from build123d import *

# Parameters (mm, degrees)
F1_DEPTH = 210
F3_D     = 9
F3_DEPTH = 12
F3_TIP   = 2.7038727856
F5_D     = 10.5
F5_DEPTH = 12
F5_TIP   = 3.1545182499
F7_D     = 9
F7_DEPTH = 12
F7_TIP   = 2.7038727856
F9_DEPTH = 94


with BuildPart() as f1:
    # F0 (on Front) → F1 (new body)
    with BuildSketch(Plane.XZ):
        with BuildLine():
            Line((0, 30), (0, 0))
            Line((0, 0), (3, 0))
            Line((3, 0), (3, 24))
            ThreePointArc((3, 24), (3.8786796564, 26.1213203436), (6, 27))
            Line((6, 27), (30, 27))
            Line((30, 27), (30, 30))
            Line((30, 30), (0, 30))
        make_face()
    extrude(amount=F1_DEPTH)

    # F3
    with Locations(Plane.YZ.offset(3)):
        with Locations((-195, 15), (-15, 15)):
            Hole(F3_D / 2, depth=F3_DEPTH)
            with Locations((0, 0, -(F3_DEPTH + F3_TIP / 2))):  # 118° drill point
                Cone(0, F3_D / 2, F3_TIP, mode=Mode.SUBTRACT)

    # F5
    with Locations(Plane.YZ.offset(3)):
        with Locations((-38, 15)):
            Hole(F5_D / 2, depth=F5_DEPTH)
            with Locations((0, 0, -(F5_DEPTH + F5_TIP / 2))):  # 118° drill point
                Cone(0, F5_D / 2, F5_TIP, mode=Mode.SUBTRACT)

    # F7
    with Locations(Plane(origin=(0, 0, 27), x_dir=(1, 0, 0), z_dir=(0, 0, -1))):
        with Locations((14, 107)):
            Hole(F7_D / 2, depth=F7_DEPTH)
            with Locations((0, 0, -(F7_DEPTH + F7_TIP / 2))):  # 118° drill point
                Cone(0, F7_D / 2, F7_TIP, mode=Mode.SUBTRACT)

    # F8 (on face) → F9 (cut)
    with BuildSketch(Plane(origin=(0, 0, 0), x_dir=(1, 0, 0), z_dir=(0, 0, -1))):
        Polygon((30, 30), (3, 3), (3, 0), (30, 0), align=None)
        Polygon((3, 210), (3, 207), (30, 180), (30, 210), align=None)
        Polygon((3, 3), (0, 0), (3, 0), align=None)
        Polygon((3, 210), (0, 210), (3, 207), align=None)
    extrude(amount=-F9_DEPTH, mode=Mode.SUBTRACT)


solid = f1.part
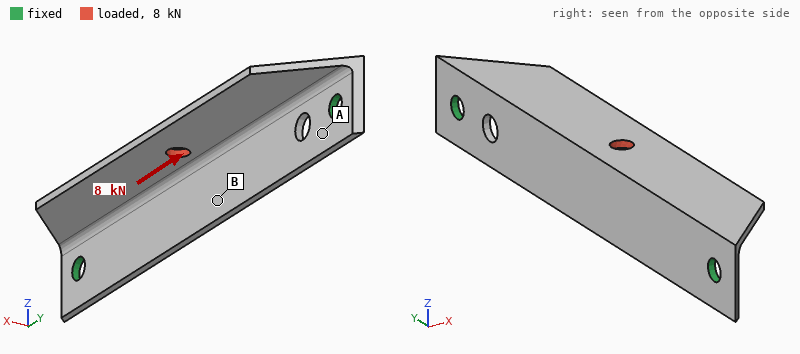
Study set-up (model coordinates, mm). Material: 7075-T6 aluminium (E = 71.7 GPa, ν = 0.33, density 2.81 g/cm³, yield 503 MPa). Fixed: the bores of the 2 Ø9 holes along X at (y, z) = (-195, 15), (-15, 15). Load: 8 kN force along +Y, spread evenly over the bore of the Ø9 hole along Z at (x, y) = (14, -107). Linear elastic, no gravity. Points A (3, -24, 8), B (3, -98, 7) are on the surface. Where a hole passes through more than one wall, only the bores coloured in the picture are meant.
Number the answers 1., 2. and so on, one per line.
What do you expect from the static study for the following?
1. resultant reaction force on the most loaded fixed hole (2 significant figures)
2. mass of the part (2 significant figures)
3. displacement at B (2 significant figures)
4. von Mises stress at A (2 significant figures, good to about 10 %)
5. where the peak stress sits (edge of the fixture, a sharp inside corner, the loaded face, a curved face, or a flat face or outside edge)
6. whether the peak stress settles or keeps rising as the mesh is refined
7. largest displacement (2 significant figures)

1. 4.3 kN
2. 91 g
3. 0.029 mm
4. 39 MPa
5. edge of the fixture
6. keeps rising
7. 0.10 mm
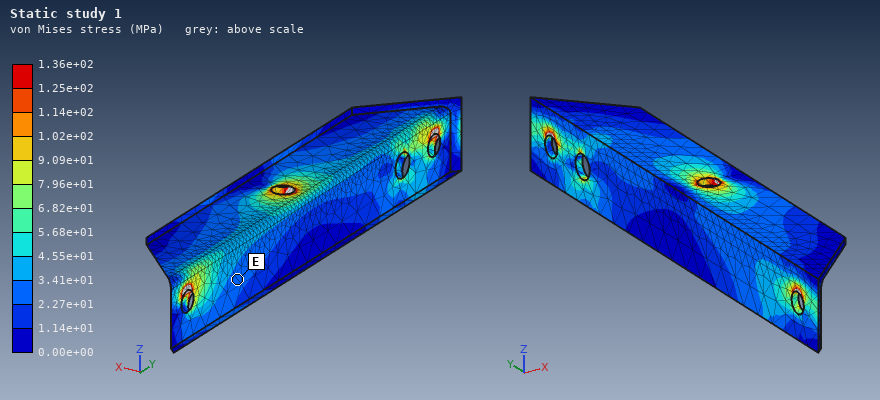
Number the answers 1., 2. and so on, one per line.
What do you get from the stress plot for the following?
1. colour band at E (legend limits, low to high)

1. 2.27e+01 to 3.41e+01 MPa
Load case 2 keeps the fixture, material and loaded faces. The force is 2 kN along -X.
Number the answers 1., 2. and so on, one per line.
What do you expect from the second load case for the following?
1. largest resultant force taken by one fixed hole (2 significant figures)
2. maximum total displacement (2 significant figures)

1. 2.0 kN
2. 0.53 mm
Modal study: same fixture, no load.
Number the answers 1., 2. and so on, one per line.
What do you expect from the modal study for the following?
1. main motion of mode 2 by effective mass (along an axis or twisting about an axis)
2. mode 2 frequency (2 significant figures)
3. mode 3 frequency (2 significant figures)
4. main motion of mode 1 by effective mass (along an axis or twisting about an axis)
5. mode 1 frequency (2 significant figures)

1. along X
2. 1700 Hz
3. 2000 Hz
4. along Z
5. 970 Hz
